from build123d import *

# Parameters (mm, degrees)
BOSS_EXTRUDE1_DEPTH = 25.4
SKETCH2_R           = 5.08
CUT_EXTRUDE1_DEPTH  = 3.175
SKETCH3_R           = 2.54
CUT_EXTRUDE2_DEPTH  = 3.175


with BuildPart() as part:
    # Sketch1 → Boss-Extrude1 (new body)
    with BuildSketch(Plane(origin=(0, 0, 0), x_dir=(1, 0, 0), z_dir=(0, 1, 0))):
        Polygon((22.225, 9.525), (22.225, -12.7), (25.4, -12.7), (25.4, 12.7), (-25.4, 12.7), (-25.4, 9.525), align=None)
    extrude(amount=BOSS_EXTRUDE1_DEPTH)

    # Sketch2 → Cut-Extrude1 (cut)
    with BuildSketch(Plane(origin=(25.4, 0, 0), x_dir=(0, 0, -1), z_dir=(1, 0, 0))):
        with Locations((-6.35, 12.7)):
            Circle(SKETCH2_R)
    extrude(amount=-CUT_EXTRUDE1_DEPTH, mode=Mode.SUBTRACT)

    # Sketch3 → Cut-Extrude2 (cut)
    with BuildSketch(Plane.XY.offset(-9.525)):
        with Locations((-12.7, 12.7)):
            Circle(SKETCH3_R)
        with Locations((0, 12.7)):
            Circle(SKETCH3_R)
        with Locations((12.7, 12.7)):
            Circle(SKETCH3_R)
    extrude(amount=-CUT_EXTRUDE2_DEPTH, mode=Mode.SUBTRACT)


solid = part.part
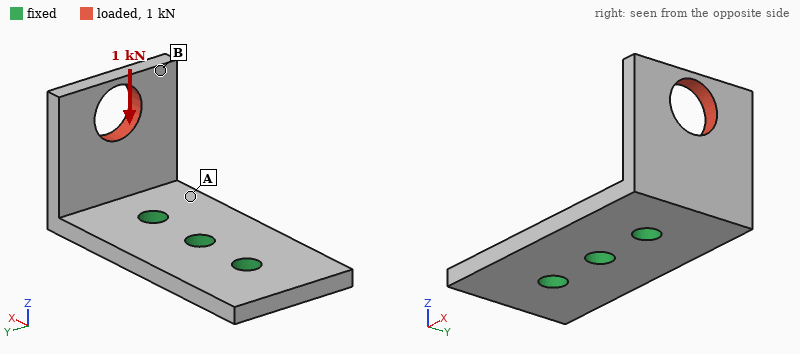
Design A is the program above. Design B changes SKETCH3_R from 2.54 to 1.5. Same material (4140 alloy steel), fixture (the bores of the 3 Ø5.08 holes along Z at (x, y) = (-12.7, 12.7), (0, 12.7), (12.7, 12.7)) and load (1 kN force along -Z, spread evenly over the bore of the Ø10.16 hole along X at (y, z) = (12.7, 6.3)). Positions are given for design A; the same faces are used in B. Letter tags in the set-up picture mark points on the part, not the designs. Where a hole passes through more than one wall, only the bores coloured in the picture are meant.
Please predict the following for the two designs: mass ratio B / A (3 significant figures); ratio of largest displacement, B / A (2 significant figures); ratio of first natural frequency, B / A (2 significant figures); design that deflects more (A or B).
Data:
1.02
1.3
0.94
B
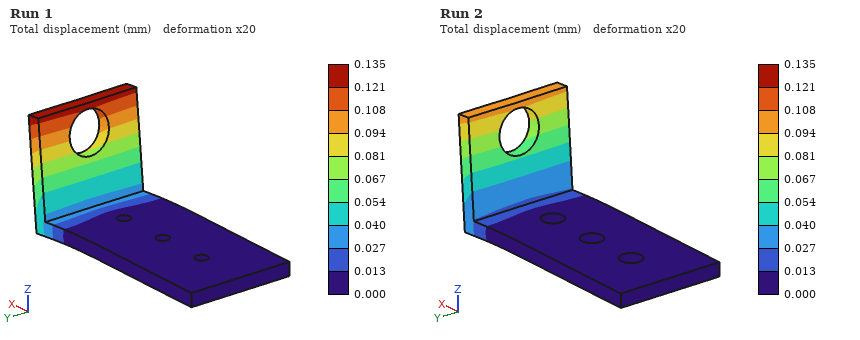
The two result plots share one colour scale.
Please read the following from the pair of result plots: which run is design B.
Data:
Run 1
